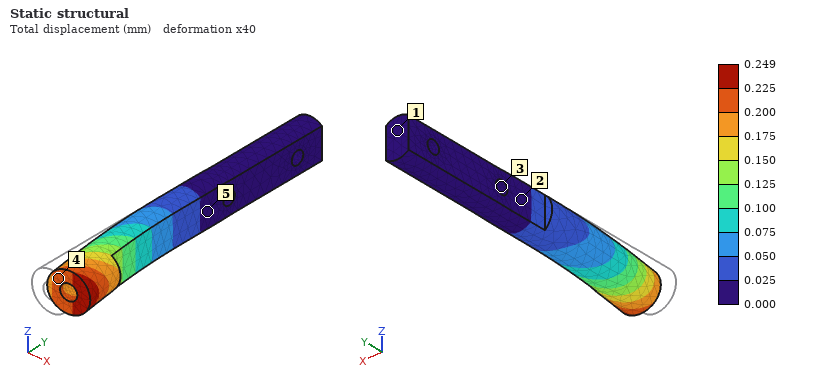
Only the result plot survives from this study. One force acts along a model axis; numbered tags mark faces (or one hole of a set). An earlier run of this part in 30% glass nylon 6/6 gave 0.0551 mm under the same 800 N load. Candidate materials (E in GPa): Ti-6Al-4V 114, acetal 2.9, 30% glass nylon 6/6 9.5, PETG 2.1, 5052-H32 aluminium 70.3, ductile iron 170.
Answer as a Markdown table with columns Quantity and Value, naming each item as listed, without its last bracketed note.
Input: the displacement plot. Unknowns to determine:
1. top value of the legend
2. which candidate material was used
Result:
| Quantity | Value |
|---|---|
| top value of the legend | 0.249 mm |
| which candidate material was used | PETG |
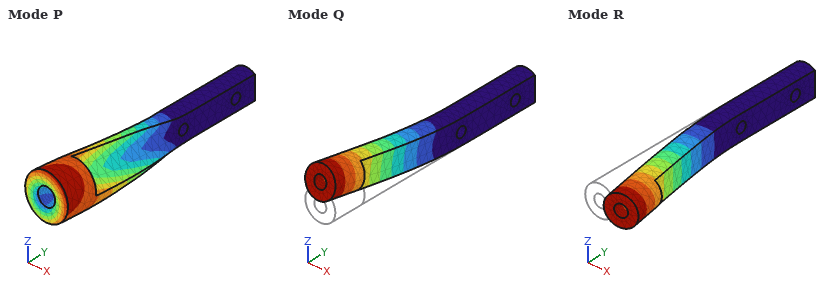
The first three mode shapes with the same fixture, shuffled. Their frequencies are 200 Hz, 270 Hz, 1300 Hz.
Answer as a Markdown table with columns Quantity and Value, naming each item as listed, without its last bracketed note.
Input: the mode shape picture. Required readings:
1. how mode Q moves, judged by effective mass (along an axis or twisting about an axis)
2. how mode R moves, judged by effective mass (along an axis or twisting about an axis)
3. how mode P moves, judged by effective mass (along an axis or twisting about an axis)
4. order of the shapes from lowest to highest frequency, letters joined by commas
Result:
| Quantity | Value |
|---|---|
| how mode Q moves, judged by effective mass | along Z |
| how mode R moves, judged by effective mass | along X |
| how mode P moves, judged by effective mass | twisting about Y |
| order of the shapes from lowest to highest frequency, letters joined by commas | R, Q, P |
